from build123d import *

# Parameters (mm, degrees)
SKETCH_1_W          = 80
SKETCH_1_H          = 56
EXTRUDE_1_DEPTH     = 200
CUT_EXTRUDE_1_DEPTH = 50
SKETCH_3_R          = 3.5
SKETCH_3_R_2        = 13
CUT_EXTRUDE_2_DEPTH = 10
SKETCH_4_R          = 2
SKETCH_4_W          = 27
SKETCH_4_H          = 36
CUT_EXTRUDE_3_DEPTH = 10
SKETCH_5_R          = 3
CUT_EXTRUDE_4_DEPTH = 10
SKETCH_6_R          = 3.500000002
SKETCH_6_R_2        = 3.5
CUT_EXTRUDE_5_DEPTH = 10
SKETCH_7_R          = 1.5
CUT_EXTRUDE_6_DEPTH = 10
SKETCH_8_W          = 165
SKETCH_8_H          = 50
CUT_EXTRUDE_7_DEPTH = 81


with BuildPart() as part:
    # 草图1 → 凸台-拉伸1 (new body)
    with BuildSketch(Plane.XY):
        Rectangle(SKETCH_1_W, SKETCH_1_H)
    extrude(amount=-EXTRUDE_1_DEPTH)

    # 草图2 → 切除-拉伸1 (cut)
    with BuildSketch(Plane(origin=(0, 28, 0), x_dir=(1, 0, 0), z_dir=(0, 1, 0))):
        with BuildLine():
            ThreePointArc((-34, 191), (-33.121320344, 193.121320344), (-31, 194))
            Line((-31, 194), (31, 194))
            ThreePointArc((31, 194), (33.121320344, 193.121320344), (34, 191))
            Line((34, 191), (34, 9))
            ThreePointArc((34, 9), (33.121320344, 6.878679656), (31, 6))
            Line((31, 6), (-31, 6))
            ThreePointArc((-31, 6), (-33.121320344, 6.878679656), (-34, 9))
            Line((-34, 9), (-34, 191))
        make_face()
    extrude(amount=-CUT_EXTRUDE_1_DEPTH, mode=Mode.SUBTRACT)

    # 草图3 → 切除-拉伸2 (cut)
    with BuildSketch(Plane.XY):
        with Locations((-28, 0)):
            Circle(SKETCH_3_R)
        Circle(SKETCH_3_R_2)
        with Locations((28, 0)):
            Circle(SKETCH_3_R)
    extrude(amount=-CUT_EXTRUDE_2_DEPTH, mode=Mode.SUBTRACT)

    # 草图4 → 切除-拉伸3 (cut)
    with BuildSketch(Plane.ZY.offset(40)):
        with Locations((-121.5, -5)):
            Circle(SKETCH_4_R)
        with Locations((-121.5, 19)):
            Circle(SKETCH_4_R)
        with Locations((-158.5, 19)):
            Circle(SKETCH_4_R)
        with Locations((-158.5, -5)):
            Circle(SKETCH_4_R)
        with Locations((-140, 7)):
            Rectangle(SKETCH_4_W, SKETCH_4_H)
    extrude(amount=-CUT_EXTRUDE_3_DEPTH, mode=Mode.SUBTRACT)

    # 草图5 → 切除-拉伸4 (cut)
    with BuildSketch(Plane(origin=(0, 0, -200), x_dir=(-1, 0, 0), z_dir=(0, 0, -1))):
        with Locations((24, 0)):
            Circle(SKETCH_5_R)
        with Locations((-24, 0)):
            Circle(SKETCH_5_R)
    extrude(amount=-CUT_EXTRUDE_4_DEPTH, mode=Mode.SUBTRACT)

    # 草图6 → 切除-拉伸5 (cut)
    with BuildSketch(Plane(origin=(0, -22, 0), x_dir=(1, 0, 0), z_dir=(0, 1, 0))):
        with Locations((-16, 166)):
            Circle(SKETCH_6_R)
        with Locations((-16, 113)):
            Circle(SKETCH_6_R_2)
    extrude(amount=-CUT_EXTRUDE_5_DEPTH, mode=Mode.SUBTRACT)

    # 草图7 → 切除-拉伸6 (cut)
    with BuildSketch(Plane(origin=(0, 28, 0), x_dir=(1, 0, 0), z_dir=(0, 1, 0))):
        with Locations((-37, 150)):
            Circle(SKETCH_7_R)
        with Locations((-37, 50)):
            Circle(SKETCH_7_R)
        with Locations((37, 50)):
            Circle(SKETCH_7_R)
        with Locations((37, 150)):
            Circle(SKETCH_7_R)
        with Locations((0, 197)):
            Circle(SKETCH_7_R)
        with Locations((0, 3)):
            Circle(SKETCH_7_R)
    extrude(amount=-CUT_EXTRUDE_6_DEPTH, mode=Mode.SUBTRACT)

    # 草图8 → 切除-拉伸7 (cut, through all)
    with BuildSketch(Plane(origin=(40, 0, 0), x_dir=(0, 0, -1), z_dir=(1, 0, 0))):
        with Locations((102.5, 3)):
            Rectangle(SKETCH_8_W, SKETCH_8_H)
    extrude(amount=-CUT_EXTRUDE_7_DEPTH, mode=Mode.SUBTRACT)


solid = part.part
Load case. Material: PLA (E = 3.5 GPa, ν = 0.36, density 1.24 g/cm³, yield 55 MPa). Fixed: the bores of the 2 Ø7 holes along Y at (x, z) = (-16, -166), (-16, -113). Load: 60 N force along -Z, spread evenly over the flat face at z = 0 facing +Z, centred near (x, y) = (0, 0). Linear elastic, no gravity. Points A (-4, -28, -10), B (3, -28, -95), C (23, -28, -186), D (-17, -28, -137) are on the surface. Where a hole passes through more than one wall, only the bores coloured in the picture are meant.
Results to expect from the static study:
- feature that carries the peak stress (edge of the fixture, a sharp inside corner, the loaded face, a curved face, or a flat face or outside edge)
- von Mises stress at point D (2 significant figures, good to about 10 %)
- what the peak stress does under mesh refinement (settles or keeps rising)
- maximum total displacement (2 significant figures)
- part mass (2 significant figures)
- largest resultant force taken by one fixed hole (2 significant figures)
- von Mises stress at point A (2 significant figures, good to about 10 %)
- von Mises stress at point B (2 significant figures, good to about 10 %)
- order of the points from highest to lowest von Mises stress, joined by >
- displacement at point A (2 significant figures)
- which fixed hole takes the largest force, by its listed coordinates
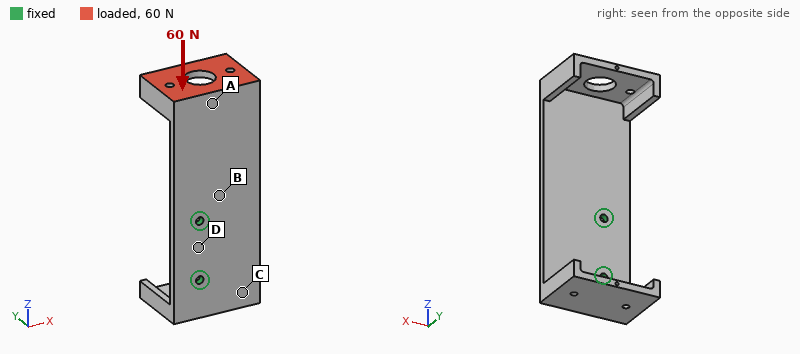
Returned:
edge of the fixture
0.65 MPa
keeps rising
2.6 mm
190 g
47 N
1.8 MPa
2.8 MPa
B > A > D > C
1.7 mm
(-16, -113)
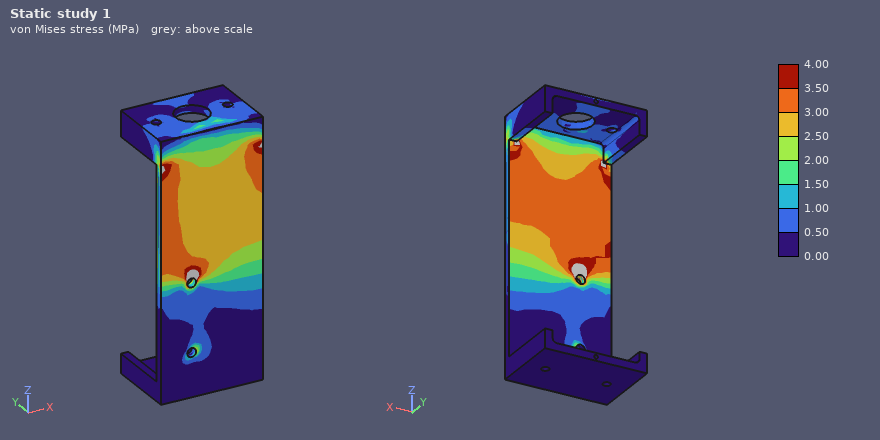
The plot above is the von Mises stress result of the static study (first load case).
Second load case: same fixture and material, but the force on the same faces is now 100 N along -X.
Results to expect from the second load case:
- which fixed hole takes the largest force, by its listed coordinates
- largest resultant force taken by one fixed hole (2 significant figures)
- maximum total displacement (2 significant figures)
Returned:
(-16, -113)
300 N
2.6 mm
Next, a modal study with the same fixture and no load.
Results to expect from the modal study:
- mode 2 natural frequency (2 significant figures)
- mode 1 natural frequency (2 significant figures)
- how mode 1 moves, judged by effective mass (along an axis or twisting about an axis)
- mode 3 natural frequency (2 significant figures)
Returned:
150 Hz
67 Hz
along Y
260 Hz
